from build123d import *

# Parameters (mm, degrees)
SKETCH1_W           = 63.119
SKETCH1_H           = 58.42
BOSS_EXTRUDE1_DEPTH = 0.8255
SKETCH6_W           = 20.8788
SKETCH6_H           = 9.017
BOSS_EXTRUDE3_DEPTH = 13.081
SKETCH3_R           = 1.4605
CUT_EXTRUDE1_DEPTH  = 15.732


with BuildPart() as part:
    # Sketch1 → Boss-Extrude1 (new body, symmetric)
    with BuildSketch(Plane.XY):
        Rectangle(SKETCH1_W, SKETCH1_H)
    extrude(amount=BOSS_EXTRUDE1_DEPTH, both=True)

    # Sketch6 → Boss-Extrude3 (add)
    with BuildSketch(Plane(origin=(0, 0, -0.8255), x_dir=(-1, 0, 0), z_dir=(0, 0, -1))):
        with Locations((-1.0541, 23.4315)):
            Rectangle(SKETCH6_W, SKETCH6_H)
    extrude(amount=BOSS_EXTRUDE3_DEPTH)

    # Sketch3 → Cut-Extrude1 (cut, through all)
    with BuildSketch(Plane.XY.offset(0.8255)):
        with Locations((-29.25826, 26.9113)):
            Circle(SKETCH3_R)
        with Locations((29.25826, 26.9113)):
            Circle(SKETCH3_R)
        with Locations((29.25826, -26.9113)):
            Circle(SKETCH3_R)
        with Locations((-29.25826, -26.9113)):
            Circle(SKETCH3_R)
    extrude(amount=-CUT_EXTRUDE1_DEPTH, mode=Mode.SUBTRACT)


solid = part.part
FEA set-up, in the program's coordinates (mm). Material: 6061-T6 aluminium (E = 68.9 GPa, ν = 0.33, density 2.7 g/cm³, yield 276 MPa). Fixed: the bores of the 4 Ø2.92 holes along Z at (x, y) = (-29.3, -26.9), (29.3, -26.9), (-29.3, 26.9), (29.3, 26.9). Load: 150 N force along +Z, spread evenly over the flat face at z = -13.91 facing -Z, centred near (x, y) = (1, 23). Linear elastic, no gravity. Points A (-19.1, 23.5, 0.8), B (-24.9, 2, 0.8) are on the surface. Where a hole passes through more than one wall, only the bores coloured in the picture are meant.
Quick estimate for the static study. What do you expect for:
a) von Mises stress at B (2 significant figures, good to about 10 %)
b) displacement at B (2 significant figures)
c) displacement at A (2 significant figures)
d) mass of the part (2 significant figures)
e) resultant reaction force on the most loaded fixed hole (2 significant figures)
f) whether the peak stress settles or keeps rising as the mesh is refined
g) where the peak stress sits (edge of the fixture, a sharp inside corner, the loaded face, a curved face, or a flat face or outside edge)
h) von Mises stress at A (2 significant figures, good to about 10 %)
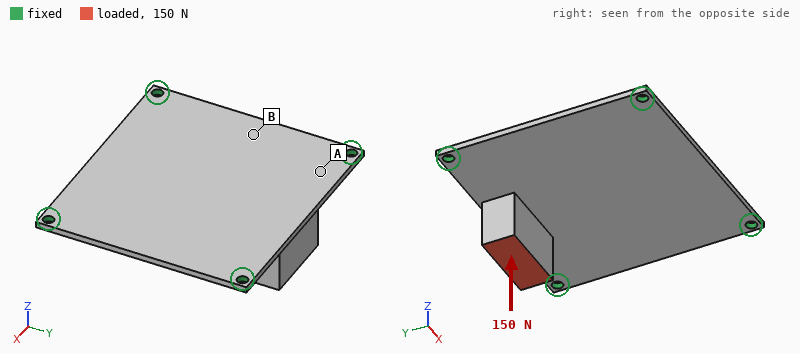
11 MPa
0.028 mm
0.066 mm
23 g
82 N
keeps rising
edge of the fixture
27 MPa
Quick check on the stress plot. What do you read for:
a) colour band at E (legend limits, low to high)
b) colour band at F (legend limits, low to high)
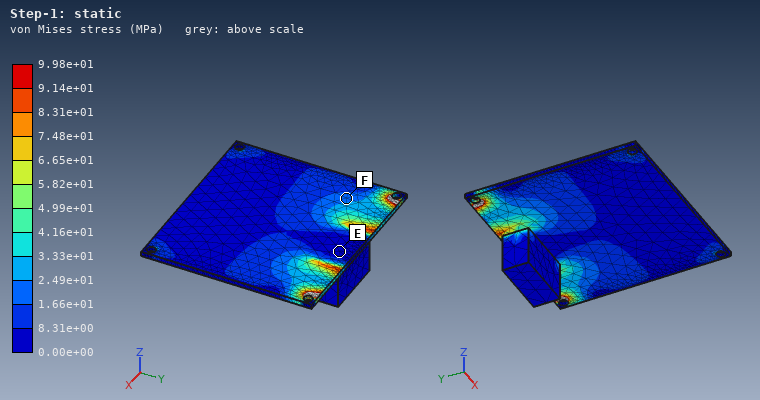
0.00e+00 to 8.31e+00 MPa
1.66e+01 to 2.49e+01 MPa
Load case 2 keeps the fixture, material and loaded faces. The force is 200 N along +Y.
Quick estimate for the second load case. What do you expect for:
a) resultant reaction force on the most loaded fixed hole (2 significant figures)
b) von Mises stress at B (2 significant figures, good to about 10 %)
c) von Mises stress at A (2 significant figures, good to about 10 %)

77 N
24 MPa
74 MPa
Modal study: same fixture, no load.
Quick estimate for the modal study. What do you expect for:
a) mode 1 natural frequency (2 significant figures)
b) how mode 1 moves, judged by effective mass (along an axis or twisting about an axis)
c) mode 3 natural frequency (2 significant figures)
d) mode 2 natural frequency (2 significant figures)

1600 Hz
along Z
3000 Hz
2000 Hz
